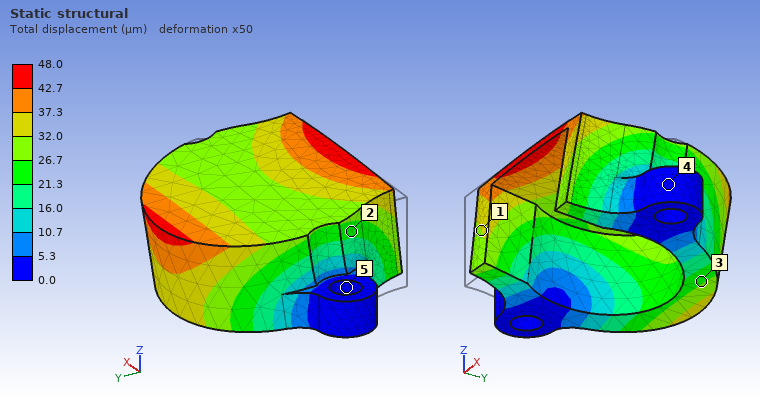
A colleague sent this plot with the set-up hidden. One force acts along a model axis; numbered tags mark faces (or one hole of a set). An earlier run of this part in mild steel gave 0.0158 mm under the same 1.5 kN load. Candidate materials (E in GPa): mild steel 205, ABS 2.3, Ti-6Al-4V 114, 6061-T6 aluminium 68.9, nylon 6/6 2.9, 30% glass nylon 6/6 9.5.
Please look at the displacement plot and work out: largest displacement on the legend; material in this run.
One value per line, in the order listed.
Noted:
48.0 µm
6061-T6 aluminium
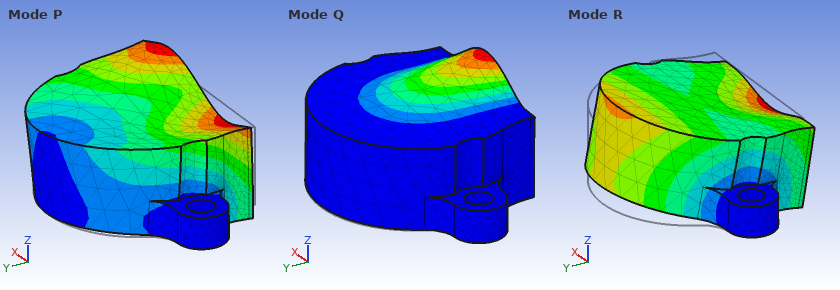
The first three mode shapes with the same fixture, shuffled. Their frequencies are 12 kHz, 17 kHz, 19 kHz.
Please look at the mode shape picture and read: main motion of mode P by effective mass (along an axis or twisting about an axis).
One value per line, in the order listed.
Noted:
along X
